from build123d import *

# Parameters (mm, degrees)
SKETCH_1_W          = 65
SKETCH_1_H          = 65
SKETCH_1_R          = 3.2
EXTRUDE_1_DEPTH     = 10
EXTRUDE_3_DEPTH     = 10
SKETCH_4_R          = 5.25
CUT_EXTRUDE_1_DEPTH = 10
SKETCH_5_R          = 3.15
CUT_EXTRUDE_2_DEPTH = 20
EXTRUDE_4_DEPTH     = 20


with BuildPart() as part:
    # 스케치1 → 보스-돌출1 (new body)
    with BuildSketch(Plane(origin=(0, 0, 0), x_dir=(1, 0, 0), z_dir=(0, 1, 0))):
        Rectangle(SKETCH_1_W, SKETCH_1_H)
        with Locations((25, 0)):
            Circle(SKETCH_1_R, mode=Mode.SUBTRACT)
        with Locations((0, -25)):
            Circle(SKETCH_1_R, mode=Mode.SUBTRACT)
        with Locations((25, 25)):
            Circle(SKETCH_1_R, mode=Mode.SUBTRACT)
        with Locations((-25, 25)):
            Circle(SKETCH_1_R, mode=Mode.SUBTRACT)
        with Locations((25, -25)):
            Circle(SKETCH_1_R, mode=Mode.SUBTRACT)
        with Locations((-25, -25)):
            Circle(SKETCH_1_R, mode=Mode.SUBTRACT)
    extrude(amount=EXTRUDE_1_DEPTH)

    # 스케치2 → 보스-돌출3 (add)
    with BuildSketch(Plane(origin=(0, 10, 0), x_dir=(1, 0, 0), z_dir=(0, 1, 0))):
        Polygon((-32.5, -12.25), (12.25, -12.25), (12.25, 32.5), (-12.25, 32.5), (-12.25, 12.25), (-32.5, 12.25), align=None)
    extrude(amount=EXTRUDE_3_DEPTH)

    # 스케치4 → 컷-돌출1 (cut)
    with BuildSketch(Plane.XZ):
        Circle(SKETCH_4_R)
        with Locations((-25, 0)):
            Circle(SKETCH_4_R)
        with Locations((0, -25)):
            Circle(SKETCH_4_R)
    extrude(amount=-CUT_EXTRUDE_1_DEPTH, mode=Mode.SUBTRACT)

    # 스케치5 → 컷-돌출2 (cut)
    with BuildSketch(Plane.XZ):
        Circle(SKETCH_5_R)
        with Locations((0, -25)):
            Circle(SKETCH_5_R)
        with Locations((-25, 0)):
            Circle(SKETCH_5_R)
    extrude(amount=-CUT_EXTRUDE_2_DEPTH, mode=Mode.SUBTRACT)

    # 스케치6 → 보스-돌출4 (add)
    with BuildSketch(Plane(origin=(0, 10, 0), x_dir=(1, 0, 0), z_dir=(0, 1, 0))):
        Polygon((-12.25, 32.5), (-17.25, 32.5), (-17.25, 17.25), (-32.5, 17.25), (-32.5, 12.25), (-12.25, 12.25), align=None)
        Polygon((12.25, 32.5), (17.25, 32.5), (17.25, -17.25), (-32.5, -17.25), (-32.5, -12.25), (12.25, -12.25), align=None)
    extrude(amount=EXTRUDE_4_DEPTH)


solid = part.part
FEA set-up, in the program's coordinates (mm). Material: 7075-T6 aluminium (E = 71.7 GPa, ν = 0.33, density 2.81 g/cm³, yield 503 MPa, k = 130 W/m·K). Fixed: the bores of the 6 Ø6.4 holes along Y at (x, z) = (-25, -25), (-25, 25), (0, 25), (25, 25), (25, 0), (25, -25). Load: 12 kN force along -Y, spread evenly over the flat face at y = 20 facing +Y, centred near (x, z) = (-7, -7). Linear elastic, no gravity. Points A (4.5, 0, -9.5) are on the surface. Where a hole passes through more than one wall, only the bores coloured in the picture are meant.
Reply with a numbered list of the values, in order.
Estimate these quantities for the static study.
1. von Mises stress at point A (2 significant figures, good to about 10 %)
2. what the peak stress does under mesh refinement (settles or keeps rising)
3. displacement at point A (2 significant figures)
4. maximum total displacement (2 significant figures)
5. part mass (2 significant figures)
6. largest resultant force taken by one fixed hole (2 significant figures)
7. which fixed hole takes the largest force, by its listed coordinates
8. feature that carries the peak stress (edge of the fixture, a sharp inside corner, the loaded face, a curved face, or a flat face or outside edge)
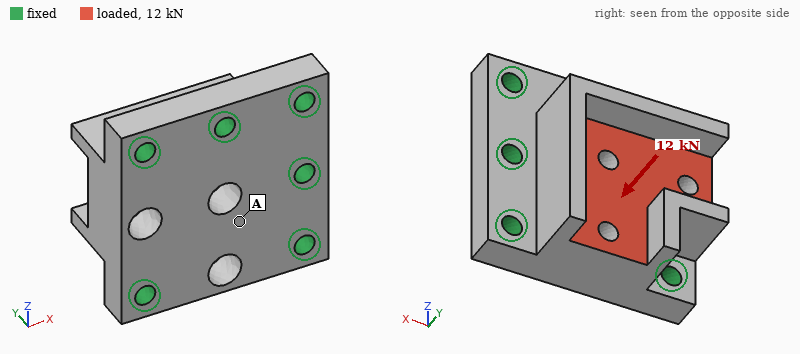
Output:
1. 12 MPa
2. keeps rising
3. 10 µm
4. 13 µm
5. 180 g
6. 5.1 kN
7. (-25, -25)
8. edge of the fixture
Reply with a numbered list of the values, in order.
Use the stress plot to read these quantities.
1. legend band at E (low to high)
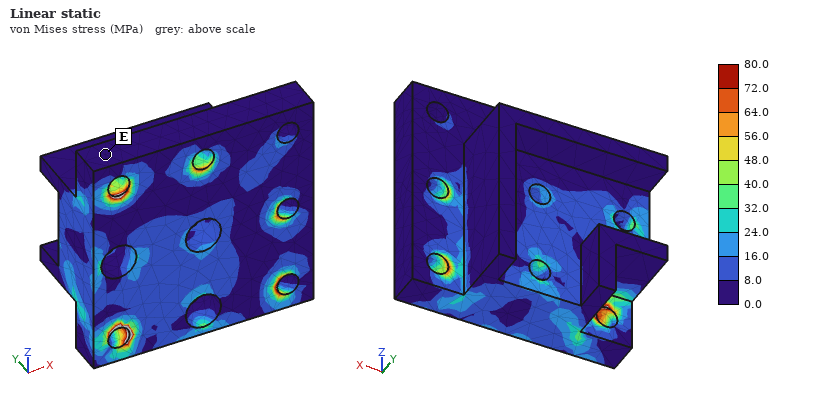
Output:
1. 0.0 to 8.0 MPa
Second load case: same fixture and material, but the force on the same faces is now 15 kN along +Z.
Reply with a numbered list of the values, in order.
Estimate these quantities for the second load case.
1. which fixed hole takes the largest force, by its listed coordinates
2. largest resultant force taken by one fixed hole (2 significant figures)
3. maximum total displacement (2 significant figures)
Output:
1. (-25, -25)
2. 4.9 kN
3. 23 µm
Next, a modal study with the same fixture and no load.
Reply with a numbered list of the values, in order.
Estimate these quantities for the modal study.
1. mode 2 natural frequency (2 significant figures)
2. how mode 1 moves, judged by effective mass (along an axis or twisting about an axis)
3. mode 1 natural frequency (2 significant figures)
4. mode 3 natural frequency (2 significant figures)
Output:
1. 17 kHz
2. along Y
3. 15 kHz
4. 20 kHz
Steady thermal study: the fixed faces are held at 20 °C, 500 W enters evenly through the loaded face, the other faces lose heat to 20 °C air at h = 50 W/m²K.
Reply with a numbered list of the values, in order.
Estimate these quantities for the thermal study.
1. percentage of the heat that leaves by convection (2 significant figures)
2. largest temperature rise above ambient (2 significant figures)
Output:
1. 4.8 %
2. 72 K
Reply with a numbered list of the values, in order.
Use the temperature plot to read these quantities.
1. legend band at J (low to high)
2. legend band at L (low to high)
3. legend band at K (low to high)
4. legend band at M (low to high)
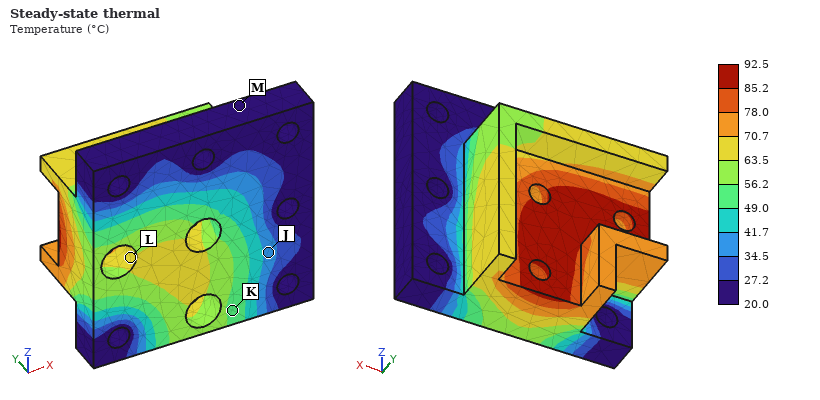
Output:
1. 34.5 to 41.7 °C
2. 63.5 to 70.7 °C
3. 49.0 to 56.2 °C
4. 20.0 to 27.2 °C
